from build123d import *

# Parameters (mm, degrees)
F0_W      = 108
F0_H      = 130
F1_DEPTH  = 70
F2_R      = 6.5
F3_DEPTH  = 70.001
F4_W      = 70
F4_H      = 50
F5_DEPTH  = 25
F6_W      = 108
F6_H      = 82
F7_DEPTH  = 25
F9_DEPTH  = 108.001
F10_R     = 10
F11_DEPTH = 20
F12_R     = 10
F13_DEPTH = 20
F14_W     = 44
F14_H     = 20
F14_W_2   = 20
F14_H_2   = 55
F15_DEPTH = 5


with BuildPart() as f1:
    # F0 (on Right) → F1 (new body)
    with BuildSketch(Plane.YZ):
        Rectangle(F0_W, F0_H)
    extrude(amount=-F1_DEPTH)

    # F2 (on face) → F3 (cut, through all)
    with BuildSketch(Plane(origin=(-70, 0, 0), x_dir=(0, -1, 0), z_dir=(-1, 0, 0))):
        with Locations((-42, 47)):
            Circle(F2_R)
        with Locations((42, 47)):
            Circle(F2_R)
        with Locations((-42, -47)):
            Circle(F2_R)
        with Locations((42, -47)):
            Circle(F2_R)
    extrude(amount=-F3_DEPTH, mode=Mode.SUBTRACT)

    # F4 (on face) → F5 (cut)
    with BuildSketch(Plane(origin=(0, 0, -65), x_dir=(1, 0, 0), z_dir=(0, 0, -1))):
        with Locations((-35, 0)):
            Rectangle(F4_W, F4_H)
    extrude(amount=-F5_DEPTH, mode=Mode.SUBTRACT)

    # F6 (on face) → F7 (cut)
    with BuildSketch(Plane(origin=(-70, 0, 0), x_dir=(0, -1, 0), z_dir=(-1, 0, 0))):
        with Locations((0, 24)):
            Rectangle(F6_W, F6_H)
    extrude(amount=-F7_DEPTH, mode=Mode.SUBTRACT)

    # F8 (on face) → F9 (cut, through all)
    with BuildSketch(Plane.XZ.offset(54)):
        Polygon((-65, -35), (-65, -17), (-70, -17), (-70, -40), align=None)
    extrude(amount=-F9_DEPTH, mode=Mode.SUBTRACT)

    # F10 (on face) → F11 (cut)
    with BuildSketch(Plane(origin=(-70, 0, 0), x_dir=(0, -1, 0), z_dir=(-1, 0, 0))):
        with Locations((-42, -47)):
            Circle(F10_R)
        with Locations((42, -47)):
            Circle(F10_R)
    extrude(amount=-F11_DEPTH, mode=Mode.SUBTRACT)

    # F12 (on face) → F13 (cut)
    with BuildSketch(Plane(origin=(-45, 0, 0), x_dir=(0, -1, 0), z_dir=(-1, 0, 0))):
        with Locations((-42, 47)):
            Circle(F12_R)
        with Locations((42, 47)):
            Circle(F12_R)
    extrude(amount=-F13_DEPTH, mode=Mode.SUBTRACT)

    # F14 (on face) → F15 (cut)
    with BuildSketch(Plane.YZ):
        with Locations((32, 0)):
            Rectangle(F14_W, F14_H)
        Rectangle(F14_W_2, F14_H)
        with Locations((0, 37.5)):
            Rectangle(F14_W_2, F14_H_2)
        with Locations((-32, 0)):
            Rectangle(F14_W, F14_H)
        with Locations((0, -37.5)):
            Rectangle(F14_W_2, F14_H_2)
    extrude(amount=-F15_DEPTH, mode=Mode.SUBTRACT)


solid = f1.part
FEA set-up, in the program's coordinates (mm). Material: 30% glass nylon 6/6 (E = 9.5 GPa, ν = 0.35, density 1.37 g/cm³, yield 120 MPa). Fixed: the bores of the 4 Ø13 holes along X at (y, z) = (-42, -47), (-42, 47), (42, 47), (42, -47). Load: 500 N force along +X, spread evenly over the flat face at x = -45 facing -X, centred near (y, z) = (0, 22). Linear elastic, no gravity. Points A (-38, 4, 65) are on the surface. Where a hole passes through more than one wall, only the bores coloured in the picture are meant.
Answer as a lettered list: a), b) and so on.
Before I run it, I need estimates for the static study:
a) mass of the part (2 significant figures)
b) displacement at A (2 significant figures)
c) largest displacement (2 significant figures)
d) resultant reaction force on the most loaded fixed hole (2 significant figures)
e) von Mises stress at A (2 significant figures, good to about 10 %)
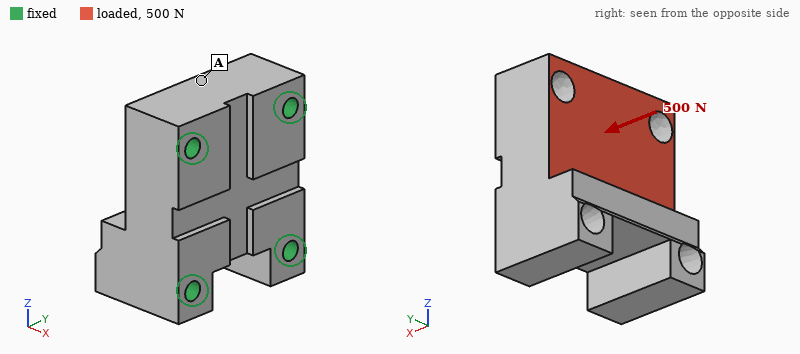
a) 820 g
b) 0.86 µm
c) 1.0 µm
d) 180 N
e) 0.069 MPa
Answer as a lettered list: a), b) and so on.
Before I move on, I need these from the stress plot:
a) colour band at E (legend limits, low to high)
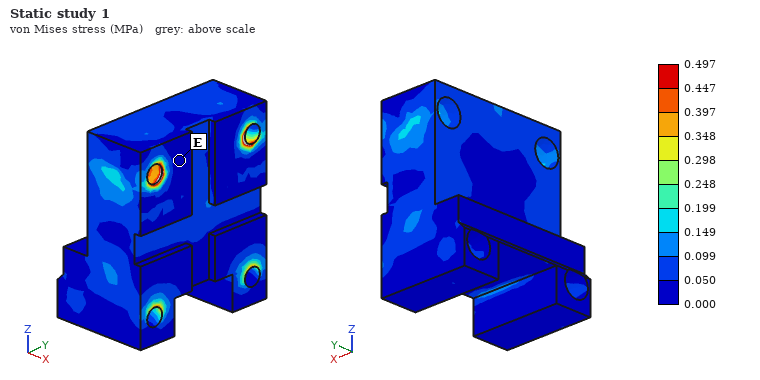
a) 0.000 to 0.050 MPa
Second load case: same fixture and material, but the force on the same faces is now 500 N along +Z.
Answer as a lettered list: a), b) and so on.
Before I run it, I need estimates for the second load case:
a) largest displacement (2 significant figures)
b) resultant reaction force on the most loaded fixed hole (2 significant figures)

a) 1.8 µm
b) 170 N
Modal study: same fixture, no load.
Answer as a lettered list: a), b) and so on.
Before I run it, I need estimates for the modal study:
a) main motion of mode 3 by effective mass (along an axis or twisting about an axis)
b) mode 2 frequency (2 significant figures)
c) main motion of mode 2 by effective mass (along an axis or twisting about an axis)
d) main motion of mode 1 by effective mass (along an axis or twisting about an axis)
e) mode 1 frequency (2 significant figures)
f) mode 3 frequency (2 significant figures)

a) along Z
b) 6300 Hz
c) along Y
d) along X
e) 5100 Hz
f) 6900 Hz
